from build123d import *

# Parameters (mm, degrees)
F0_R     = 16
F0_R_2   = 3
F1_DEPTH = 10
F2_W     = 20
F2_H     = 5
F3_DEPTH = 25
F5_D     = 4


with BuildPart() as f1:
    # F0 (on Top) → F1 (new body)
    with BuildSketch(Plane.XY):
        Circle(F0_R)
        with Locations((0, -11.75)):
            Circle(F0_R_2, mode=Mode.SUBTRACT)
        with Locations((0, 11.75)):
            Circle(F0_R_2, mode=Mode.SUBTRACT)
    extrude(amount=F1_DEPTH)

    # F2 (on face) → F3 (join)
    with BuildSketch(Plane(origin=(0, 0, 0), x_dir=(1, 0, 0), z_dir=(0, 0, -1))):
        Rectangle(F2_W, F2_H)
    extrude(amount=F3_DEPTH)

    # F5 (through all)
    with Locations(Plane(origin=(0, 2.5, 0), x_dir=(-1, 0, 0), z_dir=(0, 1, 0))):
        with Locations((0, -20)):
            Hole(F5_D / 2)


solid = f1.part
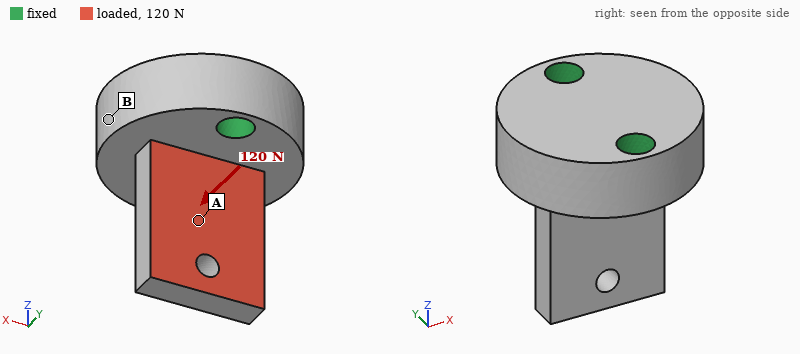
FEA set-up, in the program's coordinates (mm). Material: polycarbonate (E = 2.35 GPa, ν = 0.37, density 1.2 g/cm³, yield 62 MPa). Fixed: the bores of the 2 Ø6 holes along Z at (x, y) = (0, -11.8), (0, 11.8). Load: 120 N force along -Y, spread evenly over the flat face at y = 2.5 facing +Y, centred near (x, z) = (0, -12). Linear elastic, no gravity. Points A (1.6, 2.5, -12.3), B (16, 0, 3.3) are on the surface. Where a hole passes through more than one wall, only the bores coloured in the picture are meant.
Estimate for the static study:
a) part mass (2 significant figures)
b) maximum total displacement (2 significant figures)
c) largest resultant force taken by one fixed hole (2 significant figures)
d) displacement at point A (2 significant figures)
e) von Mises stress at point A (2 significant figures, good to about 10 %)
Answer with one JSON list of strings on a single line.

["12 g", "0.59 mm", "120 N", "0.24 mm", "4.4 MPa"]
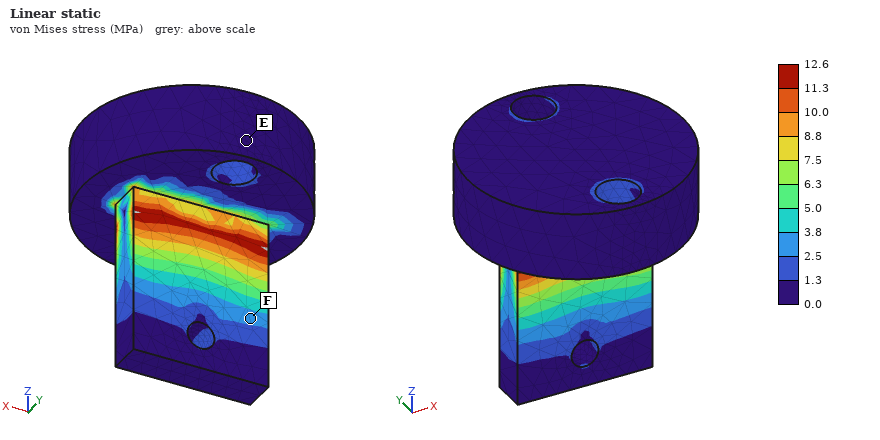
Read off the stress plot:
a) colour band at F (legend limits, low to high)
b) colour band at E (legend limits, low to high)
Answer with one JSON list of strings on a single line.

["2.5 to 3.8 MPa", "0.0 to 1.3 MPa"]
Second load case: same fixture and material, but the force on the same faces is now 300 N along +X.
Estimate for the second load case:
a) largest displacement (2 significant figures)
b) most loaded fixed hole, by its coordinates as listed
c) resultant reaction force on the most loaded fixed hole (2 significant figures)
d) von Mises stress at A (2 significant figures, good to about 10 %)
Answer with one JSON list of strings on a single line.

["0.35 mm", "(0, 11.8)", "180 N", "8.4 MPa"]
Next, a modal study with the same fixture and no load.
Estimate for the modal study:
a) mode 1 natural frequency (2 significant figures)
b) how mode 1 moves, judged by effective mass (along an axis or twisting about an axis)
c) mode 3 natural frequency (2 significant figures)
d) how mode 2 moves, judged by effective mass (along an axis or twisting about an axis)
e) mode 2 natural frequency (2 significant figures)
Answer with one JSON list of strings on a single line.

["1700 Hz", "along Y", "4100 Hz", "along X", "3400 Hz"]
